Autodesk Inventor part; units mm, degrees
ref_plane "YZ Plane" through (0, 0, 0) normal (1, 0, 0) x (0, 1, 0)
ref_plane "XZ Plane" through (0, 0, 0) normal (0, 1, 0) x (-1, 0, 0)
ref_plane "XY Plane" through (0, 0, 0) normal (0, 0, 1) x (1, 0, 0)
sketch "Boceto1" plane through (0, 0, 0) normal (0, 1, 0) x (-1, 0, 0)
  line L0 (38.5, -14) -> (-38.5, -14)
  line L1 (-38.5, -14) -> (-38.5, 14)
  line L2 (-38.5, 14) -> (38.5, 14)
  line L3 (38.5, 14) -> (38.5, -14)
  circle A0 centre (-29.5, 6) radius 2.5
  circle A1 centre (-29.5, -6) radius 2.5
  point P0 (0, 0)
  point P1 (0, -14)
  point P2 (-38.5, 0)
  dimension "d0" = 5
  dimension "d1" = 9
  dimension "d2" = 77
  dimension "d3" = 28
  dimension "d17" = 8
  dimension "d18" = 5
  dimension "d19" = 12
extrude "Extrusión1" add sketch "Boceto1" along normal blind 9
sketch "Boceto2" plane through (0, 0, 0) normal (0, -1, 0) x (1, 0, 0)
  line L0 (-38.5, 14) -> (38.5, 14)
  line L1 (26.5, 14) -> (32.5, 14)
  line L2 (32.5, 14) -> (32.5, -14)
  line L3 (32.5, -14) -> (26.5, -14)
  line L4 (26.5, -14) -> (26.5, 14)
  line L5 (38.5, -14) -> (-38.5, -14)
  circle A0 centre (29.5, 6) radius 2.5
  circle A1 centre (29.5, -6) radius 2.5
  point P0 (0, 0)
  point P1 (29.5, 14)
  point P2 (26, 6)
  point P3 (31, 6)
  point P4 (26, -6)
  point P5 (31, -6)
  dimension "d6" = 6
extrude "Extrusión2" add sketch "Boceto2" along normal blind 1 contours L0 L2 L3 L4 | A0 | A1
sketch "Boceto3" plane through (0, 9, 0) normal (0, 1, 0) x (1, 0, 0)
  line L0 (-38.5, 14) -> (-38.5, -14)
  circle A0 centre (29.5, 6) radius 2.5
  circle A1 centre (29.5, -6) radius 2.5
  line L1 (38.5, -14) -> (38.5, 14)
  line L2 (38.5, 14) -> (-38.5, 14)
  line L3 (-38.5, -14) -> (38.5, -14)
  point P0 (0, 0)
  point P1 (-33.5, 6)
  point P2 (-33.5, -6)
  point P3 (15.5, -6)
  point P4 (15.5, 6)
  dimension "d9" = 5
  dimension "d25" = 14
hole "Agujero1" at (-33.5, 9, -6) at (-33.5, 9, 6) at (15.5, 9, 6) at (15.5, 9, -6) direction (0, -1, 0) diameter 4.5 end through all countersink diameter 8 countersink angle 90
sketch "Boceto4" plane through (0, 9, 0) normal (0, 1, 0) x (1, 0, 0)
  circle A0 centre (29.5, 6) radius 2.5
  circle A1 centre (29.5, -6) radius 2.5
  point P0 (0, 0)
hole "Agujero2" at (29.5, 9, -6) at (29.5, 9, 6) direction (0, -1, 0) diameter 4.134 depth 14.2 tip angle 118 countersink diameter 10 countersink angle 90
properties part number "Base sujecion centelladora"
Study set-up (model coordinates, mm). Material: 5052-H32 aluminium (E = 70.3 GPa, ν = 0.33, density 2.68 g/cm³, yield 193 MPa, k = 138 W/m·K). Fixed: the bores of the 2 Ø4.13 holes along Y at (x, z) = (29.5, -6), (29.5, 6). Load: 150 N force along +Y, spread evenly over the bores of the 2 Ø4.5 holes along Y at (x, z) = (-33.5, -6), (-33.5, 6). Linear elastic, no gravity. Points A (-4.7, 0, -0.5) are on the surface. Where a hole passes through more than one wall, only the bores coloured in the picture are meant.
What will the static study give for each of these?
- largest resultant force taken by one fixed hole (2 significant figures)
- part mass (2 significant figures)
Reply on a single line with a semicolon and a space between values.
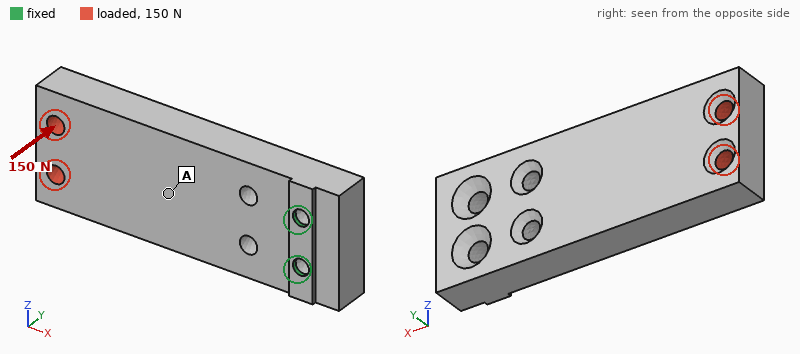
120 N; 49 g
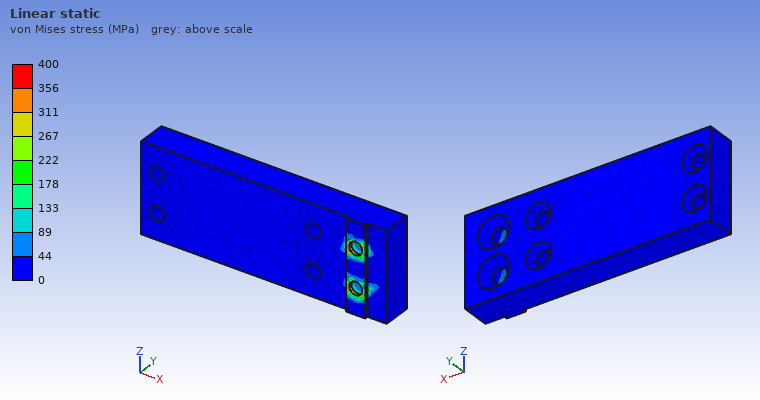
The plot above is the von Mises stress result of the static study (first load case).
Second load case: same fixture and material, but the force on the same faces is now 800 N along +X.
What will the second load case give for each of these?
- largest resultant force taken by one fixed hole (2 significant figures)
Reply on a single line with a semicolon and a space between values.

400 N
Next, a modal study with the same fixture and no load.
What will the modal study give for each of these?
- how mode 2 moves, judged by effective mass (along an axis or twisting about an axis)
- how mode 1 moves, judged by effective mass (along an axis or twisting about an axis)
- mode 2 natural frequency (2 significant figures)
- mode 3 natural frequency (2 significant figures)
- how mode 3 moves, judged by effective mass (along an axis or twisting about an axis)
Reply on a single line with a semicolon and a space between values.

along Z; along Y; 2200 Hz; 5700 Hz; twisting about X
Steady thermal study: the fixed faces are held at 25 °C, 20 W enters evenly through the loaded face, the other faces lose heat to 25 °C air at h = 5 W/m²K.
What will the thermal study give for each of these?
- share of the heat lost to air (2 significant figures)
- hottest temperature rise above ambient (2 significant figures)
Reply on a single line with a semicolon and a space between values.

4.0 %; 47 K
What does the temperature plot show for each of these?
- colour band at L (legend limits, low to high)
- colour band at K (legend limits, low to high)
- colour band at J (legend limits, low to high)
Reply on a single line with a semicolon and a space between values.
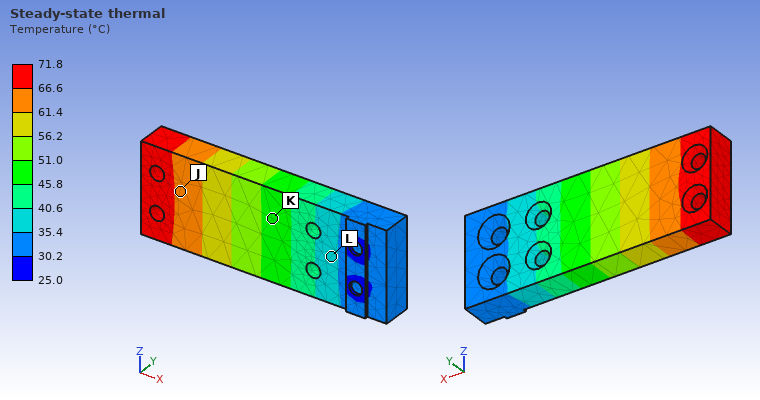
35.4 to 40.6 °C; 45.8 to 51.0 °C; 61.4 to 66.6 °C
